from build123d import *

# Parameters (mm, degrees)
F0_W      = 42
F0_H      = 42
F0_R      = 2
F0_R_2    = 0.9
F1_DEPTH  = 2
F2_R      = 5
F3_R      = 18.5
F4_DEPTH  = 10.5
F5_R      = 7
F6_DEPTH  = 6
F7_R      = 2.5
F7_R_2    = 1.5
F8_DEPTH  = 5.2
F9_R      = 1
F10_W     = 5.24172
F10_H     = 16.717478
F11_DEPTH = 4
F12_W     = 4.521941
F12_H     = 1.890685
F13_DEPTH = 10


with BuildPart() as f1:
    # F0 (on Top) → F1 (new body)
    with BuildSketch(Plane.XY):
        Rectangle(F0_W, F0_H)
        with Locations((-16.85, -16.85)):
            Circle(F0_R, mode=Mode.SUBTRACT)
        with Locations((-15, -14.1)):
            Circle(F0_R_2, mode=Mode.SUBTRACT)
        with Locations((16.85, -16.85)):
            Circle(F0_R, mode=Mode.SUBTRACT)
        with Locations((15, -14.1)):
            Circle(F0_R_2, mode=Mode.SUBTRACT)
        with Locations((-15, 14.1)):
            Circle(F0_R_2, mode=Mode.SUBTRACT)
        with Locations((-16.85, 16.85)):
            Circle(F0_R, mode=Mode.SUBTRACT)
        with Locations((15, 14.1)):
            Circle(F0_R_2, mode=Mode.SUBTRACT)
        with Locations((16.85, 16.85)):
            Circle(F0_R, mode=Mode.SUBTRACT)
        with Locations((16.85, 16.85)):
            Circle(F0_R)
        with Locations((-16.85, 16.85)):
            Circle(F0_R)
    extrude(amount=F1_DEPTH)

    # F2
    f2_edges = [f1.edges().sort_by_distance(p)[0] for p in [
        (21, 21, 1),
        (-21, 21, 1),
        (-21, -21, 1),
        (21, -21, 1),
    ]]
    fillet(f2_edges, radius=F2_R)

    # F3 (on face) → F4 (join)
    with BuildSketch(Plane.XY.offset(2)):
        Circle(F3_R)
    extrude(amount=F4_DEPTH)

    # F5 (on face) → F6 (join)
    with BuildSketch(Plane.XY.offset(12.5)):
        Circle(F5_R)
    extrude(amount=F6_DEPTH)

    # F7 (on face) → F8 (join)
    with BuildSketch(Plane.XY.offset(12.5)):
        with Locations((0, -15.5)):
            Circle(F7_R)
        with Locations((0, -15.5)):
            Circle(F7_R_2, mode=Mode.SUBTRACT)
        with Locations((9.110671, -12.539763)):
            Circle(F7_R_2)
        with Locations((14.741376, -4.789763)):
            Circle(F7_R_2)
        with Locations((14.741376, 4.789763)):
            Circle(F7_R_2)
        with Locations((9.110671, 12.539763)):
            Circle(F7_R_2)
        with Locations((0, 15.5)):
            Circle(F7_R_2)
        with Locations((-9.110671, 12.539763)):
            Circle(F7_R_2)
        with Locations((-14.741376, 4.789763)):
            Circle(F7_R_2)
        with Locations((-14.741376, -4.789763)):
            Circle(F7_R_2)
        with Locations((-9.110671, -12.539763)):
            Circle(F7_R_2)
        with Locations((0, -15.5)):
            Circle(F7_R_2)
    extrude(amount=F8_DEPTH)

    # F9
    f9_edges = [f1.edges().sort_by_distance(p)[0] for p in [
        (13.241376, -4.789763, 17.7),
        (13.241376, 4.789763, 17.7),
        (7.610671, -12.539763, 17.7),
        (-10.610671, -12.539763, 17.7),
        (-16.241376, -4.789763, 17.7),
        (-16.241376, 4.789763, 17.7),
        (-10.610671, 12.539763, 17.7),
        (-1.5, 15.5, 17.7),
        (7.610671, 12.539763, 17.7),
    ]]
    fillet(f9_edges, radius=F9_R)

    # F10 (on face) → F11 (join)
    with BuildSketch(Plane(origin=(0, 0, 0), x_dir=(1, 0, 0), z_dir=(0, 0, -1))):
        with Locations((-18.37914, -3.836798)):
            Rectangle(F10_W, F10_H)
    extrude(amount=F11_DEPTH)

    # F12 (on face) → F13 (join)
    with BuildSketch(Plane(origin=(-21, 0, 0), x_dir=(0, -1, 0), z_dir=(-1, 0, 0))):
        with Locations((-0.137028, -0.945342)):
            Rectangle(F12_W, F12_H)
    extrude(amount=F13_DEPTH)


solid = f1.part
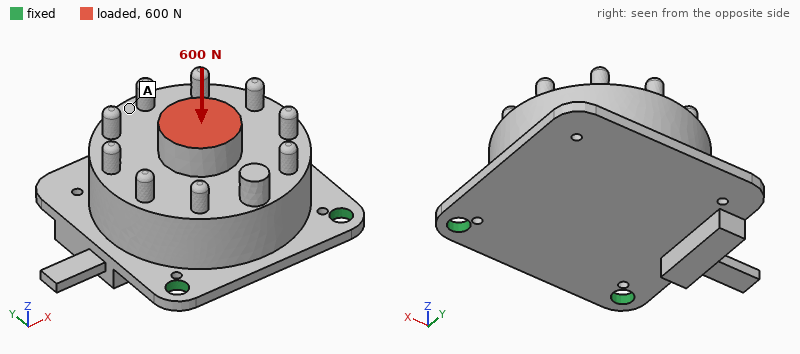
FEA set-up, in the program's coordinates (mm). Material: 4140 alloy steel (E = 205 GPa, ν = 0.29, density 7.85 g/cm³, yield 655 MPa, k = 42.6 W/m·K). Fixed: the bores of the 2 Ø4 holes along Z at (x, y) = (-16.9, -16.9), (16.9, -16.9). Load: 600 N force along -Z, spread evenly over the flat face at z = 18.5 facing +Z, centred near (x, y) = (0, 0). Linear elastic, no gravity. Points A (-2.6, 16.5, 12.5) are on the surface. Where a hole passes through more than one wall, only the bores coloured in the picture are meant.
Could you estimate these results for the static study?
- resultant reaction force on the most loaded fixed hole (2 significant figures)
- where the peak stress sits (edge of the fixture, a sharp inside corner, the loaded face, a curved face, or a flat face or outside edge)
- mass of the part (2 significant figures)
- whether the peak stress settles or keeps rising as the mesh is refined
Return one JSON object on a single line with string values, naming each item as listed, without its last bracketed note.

{"resultant reaction force on the most loaded fixed hole": "300 N", "where the peak stress sits": "edge of the fixture", "mass of the part": "130 g", "whether the peak stress settles or keeps rising as the mesh is refined": "keeps rising"}
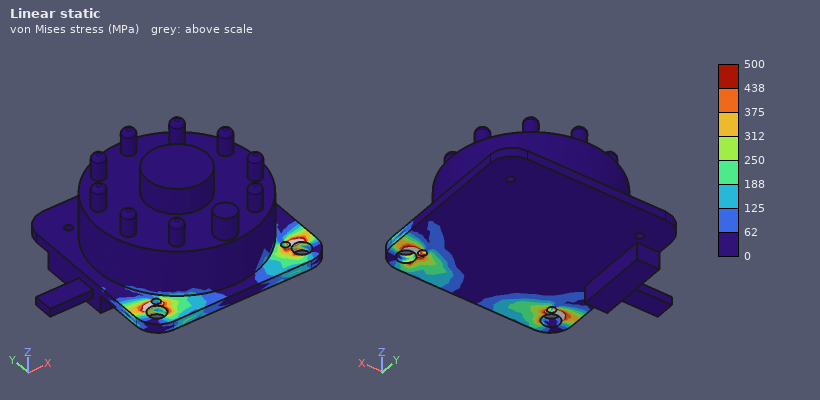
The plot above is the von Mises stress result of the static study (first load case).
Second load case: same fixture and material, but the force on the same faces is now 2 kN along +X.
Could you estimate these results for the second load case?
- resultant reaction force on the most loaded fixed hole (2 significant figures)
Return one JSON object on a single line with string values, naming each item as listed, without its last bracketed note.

{"resultant reaction force on the most loaded fixed hole": "1.8 kN"}
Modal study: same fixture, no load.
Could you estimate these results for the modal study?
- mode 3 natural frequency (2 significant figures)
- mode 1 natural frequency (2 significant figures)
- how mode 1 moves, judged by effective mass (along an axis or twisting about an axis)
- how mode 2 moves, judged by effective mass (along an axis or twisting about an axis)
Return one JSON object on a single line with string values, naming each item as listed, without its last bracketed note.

{"mode 3 natural frequency": "8300 Hz", "mode 1 natural frequency": "780 Hz", "how mode 1 moves, judged by effective mass": "along Z", "how mode 2 moves, judged by effective mass": "along X"}
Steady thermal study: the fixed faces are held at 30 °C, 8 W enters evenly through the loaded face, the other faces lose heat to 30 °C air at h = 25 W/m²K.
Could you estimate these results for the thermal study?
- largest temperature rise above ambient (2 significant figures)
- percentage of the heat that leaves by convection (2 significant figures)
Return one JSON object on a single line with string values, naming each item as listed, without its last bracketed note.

{"largest temperature rise above ambient": "32 K", "percentage of the heat that leaves by convection": "34 %"}
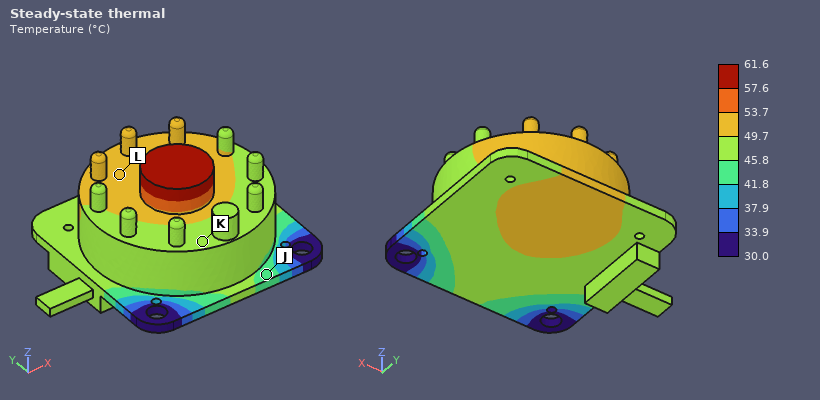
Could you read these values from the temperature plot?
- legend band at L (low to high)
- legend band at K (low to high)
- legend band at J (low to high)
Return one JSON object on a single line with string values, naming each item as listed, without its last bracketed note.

{"legend band at L": "49.7 to 53.7 °C", "legend band at K": "45.8 to 49.7 °C", "legend band at J": "41.8 to 45.8 °C"}
